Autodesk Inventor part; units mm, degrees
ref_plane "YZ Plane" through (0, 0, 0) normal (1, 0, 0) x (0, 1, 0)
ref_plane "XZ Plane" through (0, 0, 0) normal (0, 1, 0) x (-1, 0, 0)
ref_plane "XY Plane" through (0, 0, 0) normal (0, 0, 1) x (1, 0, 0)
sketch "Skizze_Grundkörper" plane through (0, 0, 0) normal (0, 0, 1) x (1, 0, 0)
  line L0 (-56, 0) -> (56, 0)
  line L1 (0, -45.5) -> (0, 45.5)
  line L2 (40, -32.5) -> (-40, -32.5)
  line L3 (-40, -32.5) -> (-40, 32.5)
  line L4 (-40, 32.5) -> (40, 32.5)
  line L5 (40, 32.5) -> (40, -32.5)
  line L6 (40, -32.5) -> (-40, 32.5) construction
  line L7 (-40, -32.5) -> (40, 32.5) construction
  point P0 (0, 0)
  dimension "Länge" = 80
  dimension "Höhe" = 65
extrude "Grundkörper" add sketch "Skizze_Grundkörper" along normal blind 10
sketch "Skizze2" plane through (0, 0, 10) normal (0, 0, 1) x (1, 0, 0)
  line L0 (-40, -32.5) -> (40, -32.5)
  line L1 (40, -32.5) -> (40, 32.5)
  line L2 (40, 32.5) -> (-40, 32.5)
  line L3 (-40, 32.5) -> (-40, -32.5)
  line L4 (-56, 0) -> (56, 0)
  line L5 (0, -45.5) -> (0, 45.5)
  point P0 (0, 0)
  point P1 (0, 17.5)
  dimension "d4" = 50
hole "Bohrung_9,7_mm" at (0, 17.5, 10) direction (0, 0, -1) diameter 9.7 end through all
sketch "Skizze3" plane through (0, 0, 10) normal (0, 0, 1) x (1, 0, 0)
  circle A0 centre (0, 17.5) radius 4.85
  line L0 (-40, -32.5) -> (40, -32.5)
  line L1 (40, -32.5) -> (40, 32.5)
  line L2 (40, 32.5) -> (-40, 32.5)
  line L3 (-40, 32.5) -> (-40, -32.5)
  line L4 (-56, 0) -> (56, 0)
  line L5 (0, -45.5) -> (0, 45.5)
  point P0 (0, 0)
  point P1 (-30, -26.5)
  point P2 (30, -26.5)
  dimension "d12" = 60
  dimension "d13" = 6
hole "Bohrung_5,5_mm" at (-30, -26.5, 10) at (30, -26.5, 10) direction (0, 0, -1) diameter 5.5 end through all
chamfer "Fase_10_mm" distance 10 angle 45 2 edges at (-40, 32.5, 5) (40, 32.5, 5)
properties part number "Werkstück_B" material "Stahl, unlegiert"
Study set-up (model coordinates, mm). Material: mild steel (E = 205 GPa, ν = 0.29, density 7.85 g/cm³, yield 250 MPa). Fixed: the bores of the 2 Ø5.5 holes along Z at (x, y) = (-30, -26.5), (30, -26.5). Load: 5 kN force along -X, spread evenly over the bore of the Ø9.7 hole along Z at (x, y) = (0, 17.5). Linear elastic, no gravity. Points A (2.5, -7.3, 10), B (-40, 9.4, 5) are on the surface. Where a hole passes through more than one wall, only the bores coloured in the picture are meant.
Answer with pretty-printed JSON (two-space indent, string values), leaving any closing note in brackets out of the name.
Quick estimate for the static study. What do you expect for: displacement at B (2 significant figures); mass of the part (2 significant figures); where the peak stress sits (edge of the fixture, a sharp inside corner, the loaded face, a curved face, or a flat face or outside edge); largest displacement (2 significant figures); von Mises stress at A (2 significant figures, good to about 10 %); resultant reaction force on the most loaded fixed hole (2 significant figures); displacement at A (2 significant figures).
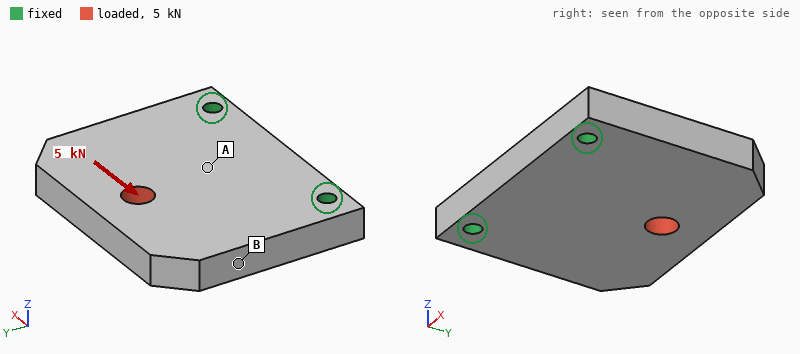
{
  "displacement at B": "6.1 µm",
  "mass of the part": "390 g",
  "where the peak stress sits": "edge of the fixture",
  "largest displacement": "8.3 µm",
  "von Mises stress at A": "15 MPa",
  "resultant reaction force on the most loaded fixed hole": "4.3 kN",
  "displacement at A": "2.8 µm"
}
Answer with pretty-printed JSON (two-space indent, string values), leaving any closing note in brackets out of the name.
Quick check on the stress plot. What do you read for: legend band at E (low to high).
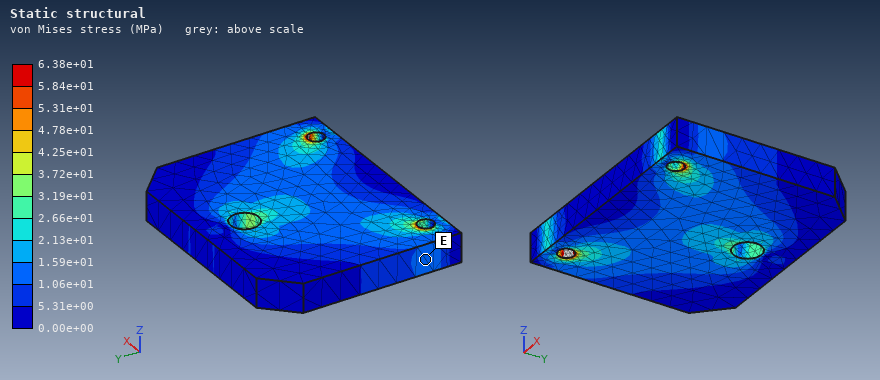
{
  "legend band at E": "1.06e+01 to 1.59e+01 MPa"
}
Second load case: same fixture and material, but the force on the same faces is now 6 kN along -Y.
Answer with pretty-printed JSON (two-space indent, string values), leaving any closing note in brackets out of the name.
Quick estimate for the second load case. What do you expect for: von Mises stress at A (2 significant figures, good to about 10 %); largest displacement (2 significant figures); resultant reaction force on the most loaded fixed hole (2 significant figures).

{
  "von Mises stress at A": "7.7 MPa",
  "largest displacement": "5.1 µm",
  "resultant reaction force on the most loaded fixed hole": "3.2 kN"
}
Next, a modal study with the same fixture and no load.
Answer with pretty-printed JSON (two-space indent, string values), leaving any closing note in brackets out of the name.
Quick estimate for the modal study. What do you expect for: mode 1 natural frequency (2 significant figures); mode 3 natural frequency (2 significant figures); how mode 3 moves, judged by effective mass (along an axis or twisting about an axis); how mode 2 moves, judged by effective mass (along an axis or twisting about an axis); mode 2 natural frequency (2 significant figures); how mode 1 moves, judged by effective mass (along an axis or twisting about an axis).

{
  "mode 1 natural frequency": "2000 Hz",
  "mode 3 natural frequency": "9400 Hz",
  "how mode 3 moves, judged by effective mass": "along X",
  "how mode 2 moves, judged by effective mass": "twisting about Y",
  "mode 2 natural frequency": "4600 Hz",
  "how mode 1 moves, judged by effective mass": "along Z"
}
